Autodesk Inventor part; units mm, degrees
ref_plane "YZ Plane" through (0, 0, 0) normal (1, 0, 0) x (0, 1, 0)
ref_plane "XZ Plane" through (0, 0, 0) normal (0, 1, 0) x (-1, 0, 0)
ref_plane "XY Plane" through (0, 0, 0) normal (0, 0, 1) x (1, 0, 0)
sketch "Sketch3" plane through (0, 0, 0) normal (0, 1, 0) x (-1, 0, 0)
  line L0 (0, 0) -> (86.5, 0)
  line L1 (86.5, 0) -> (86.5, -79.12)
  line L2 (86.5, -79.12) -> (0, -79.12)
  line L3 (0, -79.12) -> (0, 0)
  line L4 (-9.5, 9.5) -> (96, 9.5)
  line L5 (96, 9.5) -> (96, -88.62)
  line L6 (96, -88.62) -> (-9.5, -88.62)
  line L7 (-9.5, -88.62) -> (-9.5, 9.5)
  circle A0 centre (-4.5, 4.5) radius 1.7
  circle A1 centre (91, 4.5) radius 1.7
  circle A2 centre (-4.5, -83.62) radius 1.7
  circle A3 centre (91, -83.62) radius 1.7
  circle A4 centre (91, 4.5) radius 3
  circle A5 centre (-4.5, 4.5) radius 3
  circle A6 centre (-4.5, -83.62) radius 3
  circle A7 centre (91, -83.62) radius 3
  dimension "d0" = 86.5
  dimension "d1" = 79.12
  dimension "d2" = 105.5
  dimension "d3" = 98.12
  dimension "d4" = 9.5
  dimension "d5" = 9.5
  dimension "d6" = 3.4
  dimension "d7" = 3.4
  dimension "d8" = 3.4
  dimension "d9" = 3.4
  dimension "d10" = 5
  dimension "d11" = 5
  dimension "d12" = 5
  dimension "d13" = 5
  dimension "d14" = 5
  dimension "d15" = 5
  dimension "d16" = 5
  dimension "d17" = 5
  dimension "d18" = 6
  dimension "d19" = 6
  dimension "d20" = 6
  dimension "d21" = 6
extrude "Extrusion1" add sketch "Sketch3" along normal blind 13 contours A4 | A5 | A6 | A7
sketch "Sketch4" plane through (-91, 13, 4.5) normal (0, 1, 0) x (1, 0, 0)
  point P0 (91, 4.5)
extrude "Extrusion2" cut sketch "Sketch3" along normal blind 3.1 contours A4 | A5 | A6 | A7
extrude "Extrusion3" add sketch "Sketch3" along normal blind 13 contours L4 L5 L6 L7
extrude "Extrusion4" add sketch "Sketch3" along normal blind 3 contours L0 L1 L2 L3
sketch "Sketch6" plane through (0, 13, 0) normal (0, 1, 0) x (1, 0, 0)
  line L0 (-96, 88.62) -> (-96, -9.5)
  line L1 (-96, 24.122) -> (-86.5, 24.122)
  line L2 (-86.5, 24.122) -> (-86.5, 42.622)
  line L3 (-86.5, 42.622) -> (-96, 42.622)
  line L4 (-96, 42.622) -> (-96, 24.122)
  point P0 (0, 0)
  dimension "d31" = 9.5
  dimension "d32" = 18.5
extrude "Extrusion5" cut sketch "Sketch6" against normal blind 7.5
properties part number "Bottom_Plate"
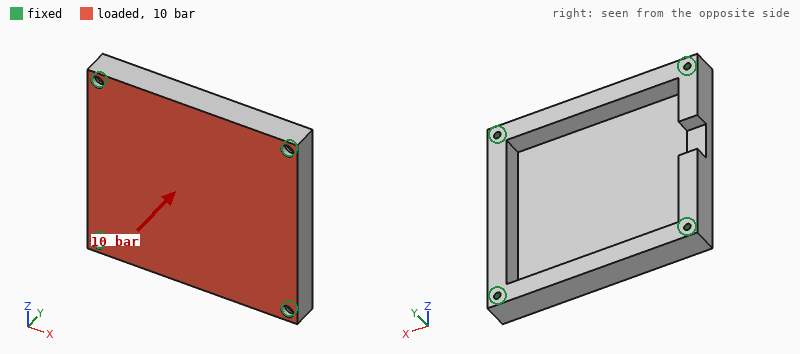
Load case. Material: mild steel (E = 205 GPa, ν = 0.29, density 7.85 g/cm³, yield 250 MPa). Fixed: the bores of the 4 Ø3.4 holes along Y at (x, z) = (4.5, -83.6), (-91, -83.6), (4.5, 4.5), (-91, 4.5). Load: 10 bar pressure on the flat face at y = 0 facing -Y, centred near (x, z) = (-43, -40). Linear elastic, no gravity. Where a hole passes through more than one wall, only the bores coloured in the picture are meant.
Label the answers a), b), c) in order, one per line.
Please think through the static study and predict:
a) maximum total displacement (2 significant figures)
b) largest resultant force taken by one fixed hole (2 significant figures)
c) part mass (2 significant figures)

a) 0.20 mm
b) 4.3 kN
c) 500 g
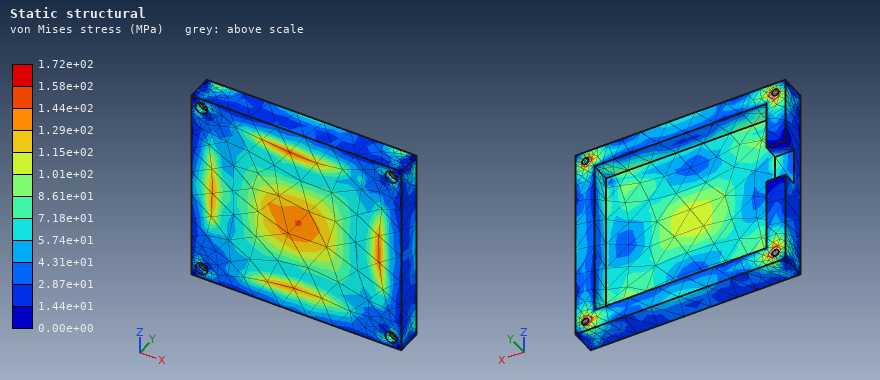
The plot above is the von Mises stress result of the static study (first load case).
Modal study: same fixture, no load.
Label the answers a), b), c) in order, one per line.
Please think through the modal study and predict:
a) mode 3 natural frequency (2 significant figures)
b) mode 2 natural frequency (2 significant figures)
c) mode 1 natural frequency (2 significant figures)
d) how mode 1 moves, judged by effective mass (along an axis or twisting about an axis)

a) 5300 Hz
b) 5100 Hz
c) 3000 Hz
d) along Y
